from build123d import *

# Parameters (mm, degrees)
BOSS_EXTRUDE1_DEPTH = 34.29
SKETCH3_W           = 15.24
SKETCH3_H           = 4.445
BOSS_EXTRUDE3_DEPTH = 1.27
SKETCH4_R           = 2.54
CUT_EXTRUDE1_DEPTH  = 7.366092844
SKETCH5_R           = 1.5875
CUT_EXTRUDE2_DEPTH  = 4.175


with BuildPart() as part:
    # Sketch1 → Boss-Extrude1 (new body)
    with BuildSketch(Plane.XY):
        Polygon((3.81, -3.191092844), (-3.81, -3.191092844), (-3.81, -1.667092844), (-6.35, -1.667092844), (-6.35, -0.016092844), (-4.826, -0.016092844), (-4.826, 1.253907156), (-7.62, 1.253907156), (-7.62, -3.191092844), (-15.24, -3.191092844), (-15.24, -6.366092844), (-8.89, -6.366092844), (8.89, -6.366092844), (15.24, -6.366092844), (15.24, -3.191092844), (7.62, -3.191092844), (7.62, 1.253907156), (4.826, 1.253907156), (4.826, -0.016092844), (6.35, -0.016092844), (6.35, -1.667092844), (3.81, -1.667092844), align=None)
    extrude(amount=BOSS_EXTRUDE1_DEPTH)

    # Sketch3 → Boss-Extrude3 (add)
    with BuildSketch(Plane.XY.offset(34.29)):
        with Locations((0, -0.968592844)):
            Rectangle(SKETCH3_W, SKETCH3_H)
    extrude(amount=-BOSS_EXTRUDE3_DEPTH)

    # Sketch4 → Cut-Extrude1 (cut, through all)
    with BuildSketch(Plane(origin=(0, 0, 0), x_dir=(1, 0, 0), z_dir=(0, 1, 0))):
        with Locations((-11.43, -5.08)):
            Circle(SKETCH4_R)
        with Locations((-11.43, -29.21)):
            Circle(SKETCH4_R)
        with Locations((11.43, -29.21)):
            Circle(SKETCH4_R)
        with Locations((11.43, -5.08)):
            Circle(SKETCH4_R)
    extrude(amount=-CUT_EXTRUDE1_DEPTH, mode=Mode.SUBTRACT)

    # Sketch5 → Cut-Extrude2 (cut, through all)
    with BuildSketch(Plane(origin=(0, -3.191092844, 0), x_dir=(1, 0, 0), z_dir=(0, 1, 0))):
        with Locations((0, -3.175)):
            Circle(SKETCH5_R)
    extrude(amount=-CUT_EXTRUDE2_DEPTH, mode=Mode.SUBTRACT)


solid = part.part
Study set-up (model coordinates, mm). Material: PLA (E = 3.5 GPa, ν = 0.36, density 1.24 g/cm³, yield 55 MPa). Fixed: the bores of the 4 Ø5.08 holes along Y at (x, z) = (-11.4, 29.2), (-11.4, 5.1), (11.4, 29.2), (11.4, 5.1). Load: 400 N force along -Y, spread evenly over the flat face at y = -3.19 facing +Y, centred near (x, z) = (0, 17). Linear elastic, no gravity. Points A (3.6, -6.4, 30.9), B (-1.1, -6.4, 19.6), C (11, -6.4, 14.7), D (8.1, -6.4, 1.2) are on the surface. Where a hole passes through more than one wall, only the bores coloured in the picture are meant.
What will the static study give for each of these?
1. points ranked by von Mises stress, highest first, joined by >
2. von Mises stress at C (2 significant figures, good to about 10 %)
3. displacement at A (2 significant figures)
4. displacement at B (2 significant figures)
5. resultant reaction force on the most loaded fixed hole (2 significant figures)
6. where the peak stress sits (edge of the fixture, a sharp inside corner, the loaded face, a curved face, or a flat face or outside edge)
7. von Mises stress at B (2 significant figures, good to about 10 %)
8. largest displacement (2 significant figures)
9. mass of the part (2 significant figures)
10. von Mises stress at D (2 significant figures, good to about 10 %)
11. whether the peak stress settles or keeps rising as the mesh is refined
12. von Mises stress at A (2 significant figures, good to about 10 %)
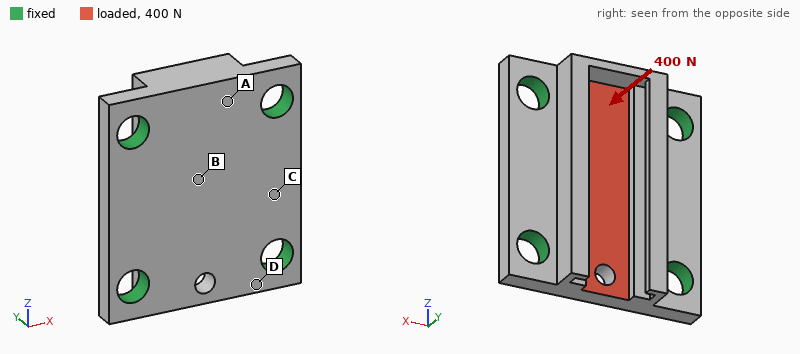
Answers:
B > D > A > C
2.7 MPa
32 µm
82 µm
100 N
edge of the fixture
12 MPa
87 µm
4.8 g
8.5 MPa
keeps rising
5.2 MPa
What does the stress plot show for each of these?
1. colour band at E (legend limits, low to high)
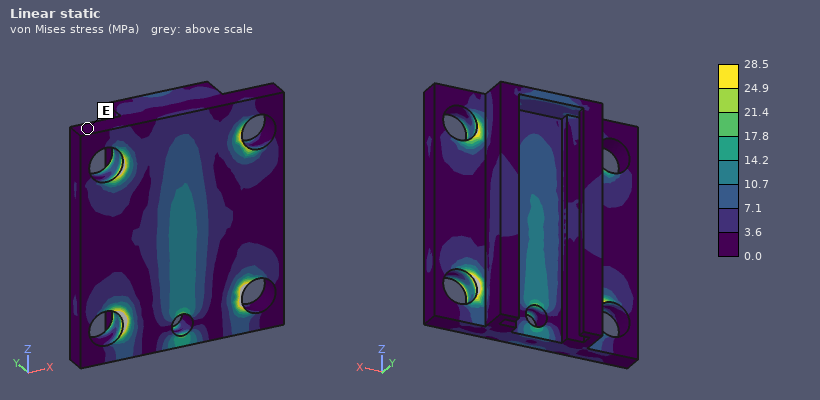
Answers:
0.0 to 3.6 MPa
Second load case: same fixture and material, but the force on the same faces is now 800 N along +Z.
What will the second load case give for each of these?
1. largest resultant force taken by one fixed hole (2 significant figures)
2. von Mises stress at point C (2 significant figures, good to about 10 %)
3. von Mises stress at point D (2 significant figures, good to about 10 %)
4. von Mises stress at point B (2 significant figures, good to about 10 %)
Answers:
210 N
2.9 MPa
3.8 MPa
1.7 MPa
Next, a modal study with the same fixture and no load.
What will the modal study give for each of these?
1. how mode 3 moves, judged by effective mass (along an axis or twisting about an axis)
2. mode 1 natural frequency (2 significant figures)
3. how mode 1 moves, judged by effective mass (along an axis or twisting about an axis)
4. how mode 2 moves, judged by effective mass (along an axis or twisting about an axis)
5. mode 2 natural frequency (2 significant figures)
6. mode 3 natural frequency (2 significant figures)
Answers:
twisting about Z
8400 Hz
along Y
twisting about X
12 kHz
13 kHz
